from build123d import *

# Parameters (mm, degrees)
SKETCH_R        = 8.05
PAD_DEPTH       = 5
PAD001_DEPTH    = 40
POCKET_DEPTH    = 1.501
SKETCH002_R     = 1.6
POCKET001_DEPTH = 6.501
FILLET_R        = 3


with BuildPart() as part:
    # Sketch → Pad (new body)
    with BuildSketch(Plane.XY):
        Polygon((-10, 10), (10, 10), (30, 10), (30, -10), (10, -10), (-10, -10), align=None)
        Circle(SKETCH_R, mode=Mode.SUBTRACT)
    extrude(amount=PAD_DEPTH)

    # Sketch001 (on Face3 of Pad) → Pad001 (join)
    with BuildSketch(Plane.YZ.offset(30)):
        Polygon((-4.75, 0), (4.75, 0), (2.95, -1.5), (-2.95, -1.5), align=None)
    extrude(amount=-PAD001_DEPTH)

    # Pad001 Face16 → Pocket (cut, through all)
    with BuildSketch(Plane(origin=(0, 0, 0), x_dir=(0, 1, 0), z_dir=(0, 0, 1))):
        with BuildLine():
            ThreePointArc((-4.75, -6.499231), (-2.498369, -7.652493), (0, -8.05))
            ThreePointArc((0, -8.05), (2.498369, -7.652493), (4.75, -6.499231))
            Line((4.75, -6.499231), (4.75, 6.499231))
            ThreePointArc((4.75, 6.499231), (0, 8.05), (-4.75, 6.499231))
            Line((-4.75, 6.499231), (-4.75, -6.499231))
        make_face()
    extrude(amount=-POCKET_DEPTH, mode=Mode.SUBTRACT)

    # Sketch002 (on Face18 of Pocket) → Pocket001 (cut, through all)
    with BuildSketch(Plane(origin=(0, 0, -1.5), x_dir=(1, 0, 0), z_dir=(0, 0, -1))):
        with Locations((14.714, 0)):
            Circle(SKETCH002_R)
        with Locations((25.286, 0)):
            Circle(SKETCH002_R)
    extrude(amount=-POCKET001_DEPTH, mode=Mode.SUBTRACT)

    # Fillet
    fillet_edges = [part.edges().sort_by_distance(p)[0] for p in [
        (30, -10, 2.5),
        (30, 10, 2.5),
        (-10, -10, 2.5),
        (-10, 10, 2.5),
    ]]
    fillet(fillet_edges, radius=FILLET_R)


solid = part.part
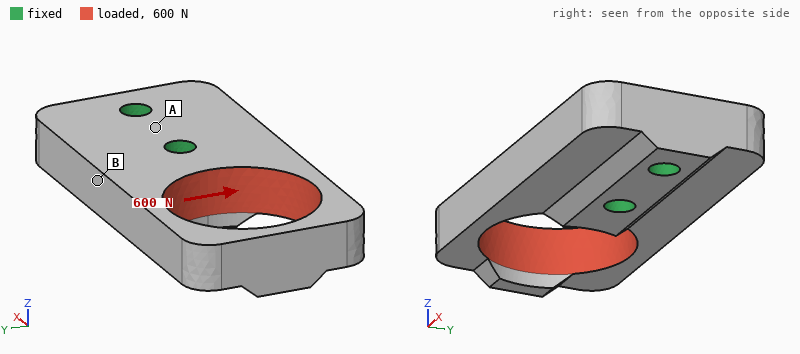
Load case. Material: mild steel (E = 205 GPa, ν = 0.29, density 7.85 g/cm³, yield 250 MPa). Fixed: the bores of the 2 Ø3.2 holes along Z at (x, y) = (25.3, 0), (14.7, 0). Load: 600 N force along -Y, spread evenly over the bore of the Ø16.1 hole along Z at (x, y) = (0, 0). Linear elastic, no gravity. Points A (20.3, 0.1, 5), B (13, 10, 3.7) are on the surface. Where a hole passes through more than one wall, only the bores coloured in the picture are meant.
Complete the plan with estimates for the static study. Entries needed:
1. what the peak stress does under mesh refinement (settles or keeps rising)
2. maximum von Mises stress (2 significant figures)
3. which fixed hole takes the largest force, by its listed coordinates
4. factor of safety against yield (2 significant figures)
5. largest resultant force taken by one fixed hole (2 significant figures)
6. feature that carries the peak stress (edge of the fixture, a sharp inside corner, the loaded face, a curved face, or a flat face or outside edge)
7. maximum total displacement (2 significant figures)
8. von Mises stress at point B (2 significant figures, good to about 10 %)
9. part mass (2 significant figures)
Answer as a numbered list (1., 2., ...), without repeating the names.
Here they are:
1. settles
2. 110 MPa
3. (14.7, 0)
4. 2.3
5. 1.2 kN
6. the loaded face
7. 27 µm
8. 34 MPa
9. 25 g
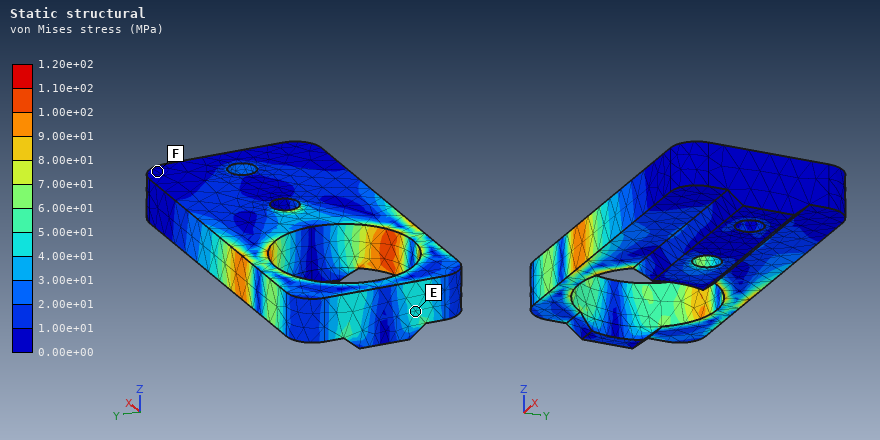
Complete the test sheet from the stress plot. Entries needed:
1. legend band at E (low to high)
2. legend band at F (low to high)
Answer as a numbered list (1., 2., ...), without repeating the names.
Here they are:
1. 4.00e+01 to 5.00e+01 MPa
2. 0.00e+00 to 1.00e+01 MPa
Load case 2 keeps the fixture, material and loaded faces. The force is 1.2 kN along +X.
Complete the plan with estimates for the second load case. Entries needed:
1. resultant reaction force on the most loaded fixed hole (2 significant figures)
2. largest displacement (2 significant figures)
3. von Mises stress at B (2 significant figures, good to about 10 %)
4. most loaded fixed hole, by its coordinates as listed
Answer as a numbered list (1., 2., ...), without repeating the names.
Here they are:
1. 730 N
2. 11 µm
3. 28 MPa
4. (14.7, 0)
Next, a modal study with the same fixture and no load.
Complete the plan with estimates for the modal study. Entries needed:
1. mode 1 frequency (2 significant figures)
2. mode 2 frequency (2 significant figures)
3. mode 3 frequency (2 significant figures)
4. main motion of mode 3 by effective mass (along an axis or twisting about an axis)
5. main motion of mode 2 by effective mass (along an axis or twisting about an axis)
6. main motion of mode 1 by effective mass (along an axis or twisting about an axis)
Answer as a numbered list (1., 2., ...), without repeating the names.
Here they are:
1. 6100 Hz
2. 9200 Hz
3. 12 kHz
4. twisting about X
5. along Y
6. along Z
